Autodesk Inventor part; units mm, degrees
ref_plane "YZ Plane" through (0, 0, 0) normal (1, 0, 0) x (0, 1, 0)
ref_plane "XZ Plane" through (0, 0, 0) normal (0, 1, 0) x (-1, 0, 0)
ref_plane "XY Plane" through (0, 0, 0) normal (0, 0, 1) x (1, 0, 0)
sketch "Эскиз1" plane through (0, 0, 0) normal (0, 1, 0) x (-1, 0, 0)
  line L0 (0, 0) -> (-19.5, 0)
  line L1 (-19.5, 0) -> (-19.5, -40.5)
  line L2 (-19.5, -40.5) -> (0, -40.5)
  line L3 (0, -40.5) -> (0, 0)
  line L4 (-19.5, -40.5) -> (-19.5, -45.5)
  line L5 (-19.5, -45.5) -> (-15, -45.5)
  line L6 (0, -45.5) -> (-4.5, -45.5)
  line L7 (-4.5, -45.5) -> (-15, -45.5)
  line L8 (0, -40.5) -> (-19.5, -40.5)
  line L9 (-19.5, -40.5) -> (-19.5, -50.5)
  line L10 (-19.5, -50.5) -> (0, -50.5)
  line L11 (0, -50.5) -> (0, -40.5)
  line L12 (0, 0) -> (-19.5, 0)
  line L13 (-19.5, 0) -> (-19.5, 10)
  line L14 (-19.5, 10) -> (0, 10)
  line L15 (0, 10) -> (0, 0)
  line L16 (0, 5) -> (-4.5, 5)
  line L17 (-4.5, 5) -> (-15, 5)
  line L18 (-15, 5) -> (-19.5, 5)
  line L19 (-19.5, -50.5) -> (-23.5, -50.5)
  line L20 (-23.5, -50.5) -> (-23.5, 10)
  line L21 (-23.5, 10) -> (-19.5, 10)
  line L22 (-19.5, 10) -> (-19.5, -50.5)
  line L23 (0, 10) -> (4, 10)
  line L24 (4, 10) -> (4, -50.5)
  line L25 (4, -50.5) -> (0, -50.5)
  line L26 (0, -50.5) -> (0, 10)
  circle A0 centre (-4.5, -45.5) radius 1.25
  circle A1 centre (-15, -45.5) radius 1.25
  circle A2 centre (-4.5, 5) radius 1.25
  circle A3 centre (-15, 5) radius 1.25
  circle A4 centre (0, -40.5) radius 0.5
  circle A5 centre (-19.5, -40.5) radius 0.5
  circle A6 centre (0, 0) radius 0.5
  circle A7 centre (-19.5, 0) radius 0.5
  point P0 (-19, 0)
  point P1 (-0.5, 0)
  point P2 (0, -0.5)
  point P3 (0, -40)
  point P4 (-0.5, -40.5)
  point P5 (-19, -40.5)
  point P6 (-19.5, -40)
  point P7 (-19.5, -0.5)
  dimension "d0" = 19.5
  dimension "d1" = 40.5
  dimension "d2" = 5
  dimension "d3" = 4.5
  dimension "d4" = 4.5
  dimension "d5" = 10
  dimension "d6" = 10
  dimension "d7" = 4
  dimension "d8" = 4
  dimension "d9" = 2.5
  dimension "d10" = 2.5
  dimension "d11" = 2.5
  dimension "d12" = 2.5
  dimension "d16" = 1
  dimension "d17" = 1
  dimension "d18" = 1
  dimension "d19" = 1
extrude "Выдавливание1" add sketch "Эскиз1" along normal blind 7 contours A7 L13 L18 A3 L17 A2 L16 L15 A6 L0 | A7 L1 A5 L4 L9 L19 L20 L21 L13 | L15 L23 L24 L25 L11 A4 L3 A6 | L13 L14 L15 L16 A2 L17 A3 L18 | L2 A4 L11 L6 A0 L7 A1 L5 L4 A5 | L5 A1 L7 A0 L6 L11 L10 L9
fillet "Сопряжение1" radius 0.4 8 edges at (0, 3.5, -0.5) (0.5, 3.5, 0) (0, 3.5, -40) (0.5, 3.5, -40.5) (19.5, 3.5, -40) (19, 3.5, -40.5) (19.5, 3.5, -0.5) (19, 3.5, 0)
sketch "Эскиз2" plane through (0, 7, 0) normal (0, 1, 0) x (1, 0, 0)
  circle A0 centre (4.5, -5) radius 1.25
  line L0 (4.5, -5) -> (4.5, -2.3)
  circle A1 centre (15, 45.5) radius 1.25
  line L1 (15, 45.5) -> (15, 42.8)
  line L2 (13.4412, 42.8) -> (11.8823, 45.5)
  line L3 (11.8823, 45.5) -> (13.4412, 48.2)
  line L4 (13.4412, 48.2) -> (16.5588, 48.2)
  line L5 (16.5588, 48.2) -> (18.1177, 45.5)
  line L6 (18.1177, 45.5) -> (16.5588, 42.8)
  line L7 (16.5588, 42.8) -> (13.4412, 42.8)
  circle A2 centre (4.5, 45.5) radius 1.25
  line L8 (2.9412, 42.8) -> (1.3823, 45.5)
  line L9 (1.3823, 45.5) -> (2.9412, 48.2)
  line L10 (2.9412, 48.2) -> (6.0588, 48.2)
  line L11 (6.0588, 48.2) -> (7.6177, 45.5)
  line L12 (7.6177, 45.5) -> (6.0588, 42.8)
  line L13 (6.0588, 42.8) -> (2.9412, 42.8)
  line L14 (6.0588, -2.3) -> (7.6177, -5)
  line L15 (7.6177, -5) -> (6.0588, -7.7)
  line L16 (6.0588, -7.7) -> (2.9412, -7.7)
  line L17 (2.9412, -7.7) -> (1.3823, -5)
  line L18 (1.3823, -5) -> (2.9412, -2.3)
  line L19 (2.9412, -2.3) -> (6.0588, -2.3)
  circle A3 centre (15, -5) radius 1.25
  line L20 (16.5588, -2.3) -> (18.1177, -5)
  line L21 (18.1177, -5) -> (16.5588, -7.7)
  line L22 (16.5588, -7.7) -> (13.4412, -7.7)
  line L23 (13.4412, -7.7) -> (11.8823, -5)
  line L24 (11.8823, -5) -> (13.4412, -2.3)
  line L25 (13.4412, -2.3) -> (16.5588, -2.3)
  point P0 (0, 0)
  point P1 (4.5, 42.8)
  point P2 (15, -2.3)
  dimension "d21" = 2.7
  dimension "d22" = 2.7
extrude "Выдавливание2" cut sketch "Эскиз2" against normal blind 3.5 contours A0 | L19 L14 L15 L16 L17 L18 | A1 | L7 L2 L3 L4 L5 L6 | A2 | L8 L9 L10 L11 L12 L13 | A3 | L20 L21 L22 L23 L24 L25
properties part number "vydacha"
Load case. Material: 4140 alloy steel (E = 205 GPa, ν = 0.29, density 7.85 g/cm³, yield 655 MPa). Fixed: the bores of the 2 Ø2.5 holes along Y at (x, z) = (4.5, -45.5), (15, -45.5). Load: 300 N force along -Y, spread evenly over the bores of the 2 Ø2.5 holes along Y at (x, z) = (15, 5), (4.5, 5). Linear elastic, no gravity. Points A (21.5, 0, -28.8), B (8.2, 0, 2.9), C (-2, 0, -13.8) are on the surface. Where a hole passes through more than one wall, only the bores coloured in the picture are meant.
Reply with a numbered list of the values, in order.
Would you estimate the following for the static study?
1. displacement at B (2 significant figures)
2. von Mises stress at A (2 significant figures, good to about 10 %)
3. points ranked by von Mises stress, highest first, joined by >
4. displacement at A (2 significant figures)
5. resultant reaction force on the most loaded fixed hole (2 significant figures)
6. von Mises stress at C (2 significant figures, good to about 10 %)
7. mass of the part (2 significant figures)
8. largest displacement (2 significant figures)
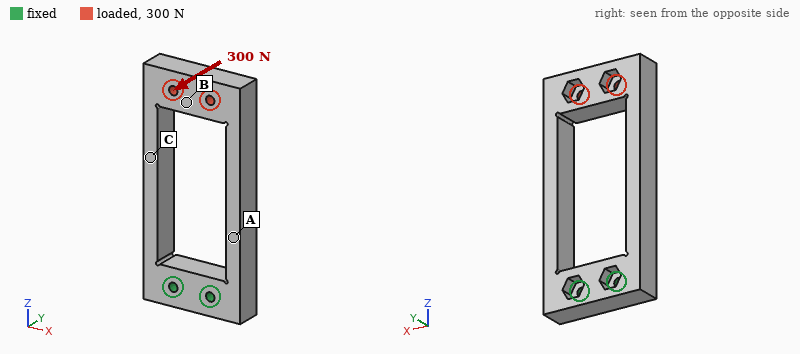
1. 0.35 mm
2. 160 MPa
3. A > C > B
4. 0.074 mm
5. 200 N
6. 87 MPa
7. 45 g
8. 0.42 mm
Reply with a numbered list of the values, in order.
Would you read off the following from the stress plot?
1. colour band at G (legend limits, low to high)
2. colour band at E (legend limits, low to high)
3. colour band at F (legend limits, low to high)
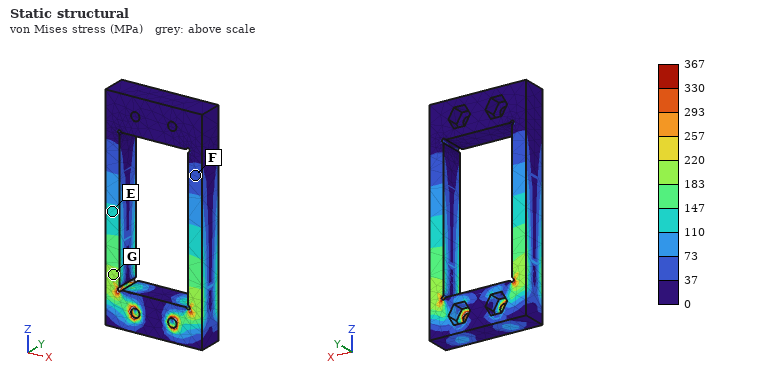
1. 183 to 220 MPa
2. 110 to 147 MPa
3. 37 to 73 MPa
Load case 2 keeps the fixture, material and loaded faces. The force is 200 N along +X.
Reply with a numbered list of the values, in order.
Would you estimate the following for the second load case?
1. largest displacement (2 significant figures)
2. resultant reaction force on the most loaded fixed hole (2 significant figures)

1. 0.15 mm
2. 730 N
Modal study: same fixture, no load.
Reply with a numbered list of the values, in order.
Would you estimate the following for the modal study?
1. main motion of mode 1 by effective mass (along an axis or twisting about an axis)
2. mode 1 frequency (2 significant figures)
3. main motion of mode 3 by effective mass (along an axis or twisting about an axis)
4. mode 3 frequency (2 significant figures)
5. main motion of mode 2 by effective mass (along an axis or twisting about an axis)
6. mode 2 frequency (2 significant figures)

1. along Y
2. 1100 Hz
3. twisting about Z
4. 3100 Hz
5. along X
6. 1400 Hz
